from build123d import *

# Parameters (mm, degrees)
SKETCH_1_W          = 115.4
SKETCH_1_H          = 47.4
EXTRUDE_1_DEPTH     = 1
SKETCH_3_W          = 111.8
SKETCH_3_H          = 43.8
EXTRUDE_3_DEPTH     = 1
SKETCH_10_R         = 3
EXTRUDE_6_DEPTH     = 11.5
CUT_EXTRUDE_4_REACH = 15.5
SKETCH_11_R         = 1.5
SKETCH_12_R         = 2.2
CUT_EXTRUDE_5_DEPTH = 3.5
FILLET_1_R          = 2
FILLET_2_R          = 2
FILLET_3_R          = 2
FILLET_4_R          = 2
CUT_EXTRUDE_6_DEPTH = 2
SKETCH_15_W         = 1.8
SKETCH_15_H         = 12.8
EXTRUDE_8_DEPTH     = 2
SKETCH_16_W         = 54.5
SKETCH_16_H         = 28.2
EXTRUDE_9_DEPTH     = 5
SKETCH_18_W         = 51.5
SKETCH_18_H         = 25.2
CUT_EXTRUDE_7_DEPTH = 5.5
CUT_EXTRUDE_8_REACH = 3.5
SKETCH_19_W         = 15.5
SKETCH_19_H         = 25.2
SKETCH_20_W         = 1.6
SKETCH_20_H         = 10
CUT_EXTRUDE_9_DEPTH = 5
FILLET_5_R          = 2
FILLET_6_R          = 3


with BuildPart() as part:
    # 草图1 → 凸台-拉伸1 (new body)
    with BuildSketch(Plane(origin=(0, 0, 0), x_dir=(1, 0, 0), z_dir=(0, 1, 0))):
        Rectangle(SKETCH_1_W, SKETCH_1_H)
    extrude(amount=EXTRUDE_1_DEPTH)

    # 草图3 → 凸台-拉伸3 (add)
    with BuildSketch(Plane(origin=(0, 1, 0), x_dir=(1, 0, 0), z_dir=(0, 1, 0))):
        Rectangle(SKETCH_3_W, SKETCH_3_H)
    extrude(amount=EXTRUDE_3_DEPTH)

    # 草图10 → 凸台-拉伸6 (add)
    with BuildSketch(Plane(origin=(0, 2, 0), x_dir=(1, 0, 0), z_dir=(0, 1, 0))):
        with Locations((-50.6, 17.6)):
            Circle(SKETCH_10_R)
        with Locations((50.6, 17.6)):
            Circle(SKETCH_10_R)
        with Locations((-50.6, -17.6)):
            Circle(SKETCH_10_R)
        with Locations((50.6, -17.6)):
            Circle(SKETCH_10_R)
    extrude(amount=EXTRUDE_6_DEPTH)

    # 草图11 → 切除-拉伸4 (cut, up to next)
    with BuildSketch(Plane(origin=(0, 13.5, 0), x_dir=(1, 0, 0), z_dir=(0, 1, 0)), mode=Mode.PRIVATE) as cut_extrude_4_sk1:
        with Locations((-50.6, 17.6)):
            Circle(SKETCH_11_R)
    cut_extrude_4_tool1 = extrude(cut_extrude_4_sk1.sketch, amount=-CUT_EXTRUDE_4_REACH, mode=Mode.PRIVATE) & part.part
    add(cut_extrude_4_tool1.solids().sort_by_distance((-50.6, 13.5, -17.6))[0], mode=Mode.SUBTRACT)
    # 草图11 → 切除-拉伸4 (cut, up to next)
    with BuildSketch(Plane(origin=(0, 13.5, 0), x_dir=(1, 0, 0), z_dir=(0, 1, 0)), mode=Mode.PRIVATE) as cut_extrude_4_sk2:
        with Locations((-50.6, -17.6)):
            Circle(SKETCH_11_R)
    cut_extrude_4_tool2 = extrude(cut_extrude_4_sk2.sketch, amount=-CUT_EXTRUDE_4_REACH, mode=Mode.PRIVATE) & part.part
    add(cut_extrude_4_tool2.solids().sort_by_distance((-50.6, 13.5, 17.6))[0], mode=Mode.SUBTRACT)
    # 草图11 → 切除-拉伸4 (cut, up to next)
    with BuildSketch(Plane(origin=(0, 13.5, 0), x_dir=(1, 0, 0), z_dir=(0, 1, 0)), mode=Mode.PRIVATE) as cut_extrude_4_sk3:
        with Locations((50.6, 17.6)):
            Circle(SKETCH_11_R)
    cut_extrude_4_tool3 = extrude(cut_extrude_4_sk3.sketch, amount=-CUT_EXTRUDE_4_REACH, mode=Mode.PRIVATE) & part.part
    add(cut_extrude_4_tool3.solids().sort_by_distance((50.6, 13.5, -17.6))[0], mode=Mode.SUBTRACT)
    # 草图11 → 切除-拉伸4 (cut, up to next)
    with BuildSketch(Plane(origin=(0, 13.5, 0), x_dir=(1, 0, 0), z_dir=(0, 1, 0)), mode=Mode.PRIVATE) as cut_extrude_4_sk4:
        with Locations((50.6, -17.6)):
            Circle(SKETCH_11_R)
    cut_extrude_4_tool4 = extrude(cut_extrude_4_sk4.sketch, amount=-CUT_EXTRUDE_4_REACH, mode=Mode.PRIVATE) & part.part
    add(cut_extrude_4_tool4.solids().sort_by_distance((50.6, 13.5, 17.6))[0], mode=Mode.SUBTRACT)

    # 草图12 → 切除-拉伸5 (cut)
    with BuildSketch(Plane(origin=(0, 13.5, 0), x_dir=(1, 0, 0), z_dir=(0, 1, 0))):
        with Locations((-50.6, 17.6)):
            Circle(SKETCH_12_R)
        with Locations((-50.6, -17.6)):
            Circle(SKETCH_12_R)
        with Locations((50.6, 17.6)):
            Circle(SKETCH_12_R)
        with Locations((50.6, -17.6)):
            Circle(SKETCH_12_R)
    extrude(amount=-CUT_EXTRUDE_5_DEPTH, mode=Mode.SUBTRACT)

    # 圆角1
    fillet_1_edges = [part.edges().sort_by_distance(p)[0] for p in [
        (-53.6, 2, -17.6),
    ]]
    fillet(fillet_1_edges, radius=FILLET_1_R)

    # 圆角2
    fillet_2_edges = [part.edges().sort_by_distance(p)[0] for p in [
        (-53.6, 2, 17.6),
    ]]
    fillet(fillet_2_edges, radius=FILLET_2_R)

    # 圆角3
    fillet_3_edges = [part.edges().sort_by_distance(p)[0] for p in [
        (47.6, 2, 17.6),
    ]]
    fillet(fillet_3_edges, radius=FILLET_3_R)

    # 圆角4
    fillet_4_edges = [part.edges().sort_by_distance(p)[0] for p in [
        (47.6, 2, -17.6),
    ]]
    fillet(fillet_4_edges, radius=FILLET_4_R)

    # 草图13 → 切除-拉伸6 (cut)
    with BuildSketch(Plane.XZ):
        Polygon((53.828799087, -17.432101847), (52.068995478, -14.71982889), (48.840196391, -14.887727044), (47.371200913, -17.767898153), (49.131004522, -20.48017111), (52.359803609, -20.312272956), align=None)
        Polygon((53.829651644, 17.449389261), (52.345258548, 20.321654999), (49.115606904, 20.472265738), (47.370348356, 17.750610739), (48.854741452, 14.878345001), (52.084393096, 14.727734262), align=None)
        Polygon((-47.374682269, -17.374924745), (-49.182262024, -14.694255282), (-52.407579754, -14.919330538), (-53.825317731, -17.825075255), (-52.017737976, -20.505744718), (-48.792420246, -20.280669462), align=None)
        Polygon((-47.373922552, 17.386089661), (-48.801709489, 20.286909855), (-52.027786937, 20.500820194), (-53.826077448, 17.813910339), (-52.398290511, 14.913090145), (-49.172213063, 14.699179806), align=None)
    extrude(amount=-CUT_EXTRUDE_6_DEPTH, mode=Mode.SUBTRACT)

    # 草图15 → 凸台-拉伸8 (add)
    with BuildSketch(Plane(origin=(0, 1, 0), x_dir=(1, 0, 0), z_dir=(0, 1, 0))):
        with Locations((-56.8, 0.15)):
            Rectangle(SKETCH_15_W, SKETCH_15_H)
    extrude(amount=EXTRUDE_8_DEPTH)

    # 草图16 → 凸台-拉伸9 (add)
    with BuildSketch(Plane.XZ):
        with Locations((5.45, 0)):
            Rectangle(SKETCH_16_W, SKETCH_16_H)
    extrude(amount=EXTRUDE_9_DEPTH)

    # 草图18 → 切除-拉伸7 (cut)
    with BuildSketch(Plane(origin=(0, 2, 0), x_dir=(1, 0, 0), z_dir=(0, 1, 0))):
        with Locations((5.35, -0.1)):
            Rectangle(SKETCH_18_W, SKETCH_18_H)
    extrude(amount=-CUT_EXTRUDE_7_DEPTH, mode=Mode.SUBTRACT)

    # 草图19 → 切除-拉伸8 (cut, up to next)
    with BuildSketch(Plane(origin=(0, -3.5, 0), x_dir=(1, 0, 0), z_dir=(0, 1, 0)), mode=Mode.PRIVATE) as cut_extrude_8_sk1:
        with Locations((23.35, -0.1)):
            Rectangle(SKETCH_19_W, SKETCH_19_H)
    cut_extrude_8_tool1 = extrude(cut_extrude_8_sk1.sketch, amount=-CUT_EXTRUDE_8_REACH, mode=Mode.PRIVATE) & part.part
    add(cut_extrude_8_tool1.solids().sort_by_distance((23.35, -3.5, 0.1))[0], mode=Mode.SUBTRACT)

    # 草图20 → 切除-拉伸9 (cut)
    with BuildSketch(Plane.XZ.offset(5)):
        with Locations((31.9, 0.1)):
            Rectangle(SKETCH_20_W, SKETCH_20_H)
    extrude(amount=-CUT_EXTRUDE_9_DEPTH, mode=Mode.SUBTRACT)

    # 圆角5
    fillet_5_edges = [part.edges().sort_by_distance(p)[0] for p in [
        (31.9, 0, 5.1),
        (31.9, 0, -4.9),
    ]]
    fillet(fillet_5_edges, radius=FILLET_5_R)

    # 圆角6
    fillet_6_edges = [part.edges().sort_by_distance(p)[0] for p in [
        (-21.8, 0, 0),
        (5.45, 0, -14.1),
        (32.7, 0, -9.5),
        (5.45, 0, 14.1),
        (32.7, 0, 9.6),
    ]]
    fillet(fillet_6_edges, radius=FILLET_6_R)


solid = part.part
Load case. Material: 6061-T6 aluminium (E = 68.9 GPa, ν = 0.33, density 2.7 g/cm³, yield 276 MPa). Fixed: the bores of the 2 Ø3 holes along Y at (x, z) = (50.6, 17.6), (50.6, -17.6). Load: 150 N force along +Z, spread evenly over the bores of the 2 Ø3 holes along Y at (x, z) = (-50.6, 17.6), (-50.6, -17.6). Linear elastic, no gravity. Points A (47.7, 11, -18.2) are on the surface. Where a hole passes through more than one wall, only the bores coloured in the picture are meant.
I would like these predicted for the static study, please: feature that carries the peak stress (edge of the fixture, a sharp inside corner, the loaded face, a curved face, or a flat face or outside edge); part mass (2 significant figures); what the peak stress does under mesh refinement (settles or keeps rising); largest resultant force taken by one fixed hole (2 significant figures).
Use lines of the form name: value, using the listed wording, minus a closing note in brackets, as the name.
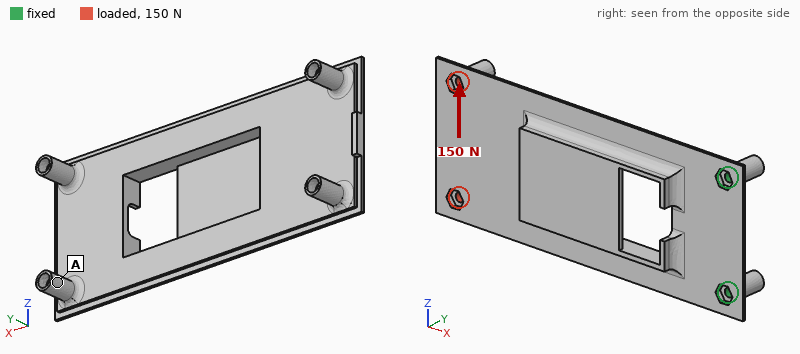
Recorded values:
feature that carries the peak stress: edge of the fixture
part mass: 31 g
what the peak stress does under mesh refinement: keeps rising
largest resultant force taken by one fixed hole: 410 N
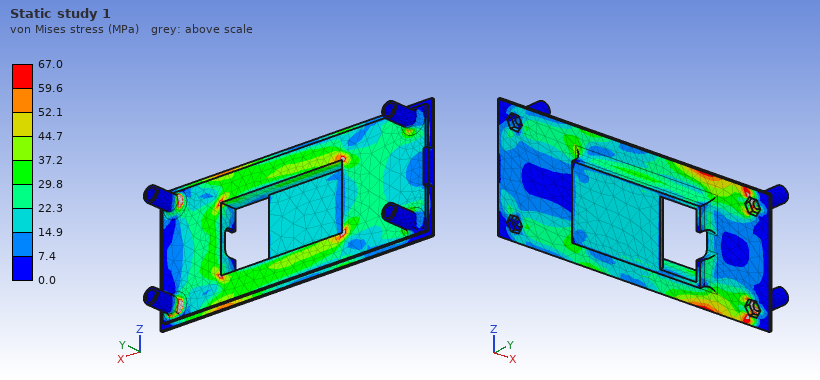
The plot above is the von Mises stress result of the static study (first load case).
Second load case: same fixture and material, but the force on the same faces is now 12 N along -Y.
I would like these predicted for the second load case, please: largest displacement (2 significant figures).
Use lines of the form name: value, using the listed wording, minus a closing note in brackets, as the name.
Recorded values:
largest displacement: 1.3 mm
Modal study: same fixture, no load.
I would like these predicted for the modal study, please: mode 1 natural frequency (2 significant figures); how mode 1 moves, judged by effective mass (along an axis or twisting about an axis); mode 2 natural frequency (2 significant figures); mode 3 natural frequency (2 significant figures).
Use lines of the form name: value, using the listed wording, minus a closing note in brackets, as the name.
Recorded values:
mode 1 natural frequency: 160 Hz
how mode 1 moves, judged by effective mass: along Y
mode 2 natural frequency: 750 Hz
mode 3 natural frequency: 1400 Hz
